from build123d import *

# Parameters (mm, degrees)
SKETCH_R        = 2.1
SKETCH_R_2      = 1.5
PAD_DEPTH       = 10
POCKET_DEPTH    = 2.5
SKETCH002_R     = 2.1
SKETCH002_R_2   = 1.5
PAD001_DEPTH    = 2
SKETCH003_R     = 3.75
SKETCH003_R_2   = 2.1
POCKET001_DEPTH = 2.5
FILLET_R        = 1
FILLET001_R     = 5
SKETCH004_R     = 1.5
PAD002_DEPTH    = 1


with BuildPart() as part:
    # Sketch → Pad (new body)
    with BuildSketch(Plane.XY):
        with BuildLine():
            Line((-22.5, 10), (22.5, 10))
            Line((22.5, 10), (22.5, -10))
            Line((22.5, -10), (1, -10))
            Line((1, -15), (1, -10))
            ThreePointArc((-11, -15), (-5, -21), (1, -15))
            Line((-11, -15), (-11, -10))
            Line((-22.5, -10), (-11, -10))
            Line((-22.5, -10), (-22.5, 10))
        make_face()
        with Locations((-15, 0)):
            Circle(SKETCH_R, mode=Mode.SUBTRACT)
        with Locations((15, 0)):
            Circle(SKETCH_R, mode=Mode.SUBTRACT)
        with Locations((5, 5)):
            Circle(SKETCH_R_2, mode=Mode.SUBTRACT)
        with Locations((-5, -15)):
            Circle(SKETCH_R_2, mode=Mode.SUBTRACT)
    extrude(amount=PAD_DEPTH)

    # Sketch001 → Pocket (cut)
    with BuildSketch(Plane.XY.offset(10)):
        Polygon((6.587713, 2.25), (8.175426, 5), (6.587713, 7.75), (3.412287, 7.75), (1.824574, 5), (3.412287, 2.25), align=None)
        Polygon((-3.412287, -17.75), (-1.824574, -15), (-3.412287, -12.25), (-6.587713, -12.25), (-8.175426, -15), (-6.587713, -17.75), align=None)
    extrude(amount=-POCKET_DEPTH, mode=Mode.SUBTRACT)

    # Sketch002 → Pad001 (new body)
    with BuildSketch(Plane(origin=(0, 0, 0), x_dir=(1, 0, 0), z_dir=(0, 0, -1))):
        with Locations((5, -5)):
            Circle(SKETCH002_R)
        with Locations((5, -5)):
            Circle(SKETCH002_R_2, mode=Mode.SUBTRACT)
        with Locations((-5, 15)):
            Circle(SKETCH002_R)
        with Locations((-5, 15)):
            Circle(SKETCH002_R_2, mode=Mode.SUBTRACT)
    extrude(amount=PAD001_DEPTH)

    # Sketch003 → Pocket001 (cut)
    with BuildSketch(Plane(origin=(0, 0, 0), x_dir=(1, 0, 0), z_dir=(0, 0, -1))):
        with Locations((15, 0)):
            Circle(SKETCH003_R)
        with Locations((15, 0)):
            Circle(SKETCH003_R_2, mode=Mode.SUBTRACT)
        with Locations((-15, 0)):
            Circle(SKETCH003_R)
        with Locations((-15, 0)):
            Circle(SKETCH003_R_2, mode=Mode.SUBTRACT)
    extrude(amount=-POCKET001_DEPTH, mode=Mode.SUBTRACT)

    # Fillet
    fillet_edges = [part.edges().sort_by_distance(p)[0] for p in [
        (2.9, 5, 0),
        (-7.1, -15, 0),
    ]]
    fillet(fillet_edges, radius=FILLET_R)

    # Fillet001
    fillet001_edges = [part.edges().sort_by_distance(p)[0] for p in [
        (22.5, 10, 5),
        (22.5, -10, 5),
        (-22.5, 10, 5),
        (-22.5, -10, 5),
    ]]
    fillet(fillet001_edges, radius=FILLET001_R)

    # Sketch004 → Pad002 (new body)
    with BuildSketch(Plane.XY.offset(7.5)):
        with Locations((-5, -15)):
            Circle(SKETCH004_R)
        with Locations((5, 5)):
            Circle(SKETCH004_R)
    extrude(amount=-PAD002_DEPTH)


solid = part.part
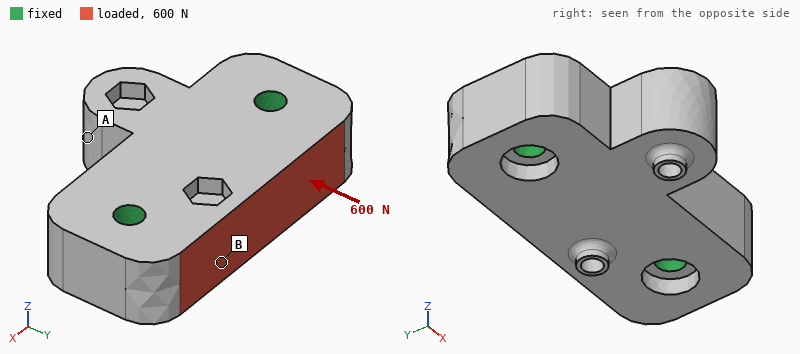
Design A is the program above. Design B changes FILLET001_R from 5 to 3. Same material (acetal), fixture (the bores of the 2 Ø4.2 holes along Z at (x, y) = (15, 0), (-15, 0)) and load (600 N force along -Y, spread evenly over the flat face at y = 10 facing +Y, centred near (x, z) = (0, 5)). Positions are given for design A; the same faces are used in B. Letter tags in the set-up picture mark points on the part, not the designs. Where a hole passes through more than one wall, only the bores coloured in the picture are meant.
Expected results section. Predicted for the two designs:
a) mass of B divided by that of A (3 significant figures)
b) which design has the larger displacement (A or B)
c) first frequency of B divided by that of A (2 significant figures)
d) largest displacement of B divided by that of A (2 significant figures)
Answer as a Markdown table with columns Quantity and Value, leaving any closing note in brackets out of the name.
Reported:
| Quantity | Value |
|---|---|
| mass of B divided by that of A | 1.01 |
| which design has the larger displacement | A |
| first frequency of B divided by that of A | 1.00 |
| largest displacement of B divided by that of A | 0.90 |
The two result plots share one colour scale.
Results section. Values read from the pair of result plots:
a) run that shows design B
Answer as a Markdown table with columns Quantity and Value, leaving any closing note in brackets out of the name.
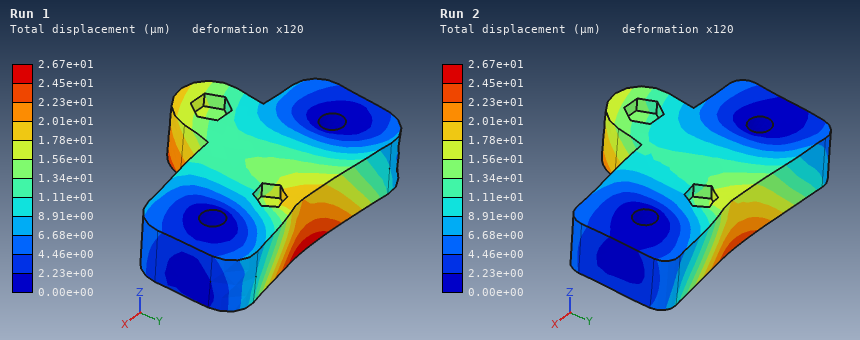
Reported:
| Quantity | Value |
|---|---|
| run that shows design B | Run 2 |
